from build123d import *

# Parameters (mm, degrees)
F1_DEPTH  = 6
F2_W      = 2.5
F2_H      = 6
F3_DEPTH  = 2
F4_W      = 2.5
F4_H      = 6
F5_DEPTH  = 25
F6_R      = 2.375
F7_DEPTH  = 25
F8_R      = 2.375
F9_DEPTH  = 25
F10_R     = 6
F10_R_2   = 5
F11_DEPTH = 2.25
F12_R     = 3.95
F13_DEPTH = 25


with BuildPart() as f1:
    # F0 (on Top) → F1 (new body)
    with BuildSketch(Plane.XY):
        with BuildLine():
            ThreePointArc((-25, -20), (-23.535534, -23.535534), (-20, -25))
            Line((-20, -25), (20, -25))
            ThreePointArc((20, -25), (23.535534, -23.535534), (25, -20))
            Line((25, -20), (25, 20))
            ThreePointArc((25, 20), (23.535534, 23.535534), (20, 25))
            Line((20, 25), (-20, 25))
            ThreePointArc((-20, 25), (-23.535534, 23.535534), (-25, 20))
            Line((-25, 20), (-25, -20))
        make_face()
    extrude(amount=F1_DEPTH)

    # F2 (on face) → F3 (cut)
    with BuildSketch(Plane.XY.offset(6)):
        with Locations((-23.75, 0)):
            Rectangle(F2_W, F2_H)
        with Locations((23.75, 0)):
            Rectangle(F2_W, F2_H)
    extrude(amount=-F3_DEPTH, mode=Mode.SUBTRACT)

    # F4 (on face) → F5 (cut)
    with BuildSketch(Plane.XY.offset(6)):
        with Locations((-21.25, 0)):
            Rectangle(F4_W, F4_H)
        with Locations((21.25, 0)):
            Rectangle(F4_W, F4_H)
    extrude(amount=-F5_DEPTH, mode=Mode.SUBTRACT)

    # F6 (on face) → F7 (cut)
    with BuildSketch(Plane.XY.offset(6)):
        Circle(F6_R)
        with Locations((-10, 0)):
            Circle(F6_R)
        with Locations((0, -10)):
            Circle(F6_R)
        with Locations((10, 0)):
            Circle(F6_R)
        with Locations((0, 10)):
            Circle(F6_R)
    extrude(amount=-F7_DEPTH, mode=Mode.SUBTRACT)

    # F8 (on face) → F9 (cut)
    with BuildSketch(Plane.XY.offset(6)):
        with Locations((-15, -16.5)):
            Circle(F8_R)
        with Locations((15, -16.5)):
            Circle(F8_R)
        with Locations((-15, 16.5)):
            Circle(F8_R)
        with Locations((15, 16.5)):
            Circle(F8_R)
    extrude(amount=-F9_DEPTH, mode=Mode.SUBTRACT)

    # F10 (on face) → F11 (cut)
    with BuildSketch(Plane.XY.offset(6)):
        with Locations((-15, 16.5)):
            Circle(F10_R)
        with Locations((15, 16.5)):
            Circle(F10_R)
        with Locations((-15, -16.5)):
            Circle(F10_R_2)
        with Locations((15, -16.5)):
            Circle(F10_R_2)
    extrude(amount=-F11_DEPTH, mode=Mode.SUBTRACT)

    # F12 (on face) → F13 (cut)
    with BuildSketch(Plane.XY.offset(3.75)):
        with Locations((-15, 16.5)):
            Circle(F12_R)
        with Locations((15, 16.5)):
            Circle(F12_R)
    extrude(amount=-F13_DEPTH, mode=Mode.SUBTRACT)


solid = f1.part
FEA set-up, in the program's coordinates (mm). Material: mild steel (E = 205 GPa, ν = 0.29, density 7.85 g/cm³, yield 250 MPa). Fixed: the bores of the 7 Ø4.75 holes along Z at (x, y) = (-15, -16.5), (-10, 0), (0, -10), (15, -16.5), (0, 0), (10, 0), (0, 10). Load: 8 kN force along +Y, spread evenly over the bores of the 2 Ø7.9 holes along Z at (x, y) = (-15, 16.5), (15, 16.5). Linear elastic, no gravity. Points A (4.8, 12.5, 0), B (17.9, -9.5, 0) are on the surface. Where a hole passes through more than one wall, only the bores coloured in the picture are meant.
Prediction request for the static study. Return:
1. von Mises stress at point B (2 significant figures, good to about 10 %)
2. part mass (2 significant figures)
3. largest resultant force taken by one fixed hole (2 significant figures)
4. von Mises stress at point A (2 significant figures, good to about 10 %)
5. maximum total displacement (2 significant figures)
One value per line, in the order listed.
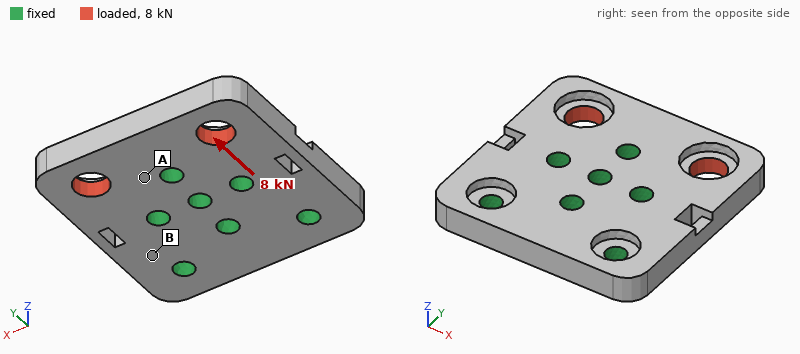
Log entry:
19 MPa
100 g
2.1 kN
46 MPa
10.0 µm
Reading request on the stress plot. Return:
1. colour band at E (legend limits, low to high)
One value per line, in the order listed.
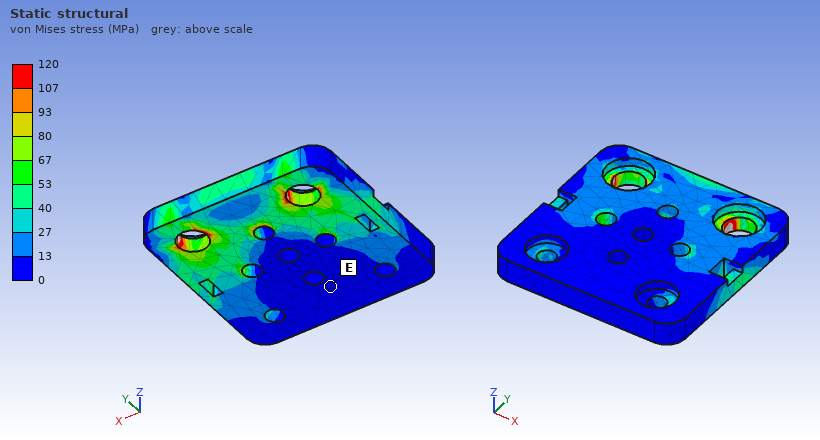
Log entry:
0 to 13 MPa
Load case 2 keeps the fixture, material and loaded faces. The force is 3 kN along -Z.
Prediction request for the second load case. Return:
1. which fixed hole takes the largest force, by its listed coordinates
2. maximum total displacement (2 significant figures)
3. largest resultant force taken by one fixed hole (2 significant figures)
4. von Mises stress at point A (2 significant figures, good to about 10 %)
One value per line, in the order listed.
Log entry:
(0, 10)
31 µm
2.1 kN
78 MPa
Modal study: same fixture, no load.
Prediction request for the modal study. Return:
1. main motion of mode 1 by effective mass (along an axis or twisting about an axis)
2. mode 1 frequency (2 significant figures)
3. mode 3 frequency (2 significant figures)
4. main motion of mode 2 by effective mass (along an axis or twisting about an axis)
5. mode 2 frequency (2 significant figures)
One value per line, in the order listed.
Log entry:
twisting about Y
11 kHz
20 kHz
along Z
12 kHz
